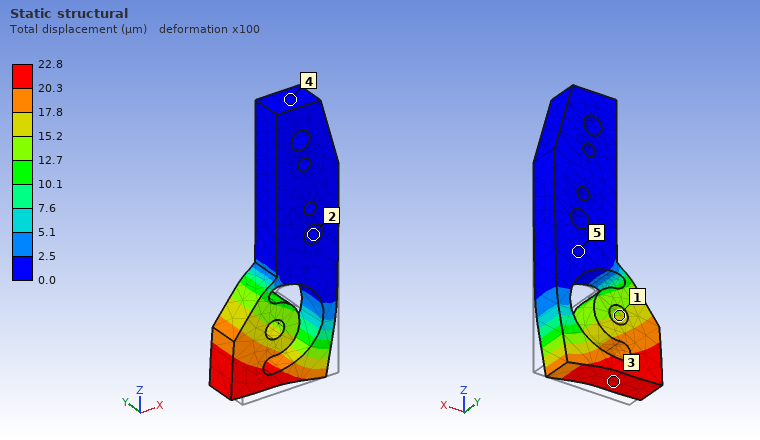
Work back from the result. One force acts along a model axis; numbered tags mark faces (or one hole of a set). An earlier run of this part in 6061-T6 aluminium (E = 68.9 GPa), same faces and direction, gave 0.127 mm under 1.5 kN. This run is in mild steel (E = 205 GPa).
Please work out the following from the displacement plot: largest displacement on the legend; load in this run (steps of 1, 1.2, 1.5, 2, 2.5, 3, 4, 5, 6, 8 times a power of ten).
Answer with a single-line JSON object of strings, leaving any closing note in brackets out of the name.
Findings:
{"largest displacement on the legend": "22.8 µm", "load in this run": "800 N"}
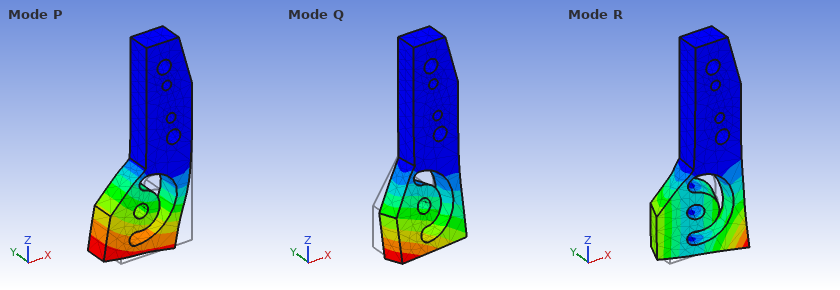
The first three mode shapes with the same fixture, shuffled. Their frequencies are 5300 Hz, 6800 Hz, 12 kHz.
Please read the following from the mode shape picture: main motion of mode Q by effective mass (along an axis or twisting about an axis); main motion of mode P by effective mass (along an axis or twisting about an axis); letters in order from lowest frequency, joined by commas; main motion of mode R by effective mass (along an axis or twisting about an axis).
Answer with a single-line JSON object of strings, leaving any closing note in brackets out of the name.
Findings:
{"main motion of mode Q by effective mass": "along Y", "main motion of mode P by effective mass": "along X", "letters in order from lowest frequency, joined by commas": "Q, P, R", "main motion of mode R by effective mass": "twisting about Z"}
